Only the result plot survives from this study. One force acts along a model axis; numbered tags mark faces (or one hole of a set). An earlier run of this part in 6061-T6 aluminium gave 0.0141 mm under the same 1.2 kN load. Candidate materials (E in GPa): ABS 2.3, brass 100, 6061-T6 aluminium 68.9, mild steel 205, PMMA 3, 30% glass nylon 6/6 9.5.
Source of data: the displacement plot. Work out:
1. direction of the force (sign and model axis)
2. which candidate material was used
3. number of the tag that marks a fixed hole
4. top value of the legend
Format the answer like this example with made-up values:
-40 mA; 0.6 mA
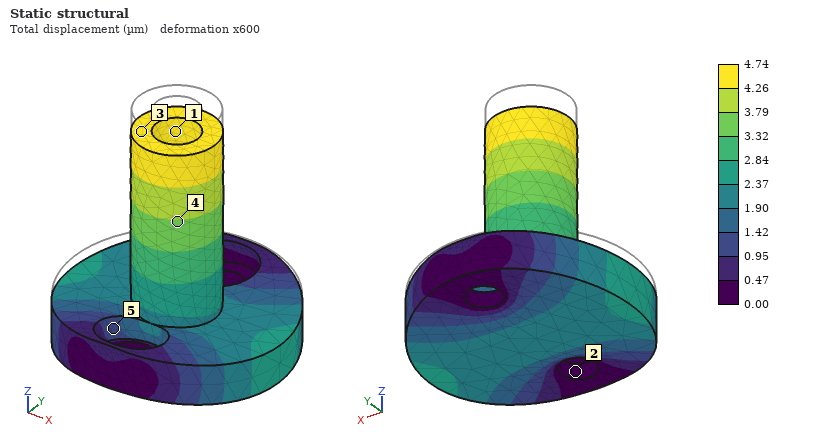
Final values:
-Z; mild steel; 2; 4.74 µm
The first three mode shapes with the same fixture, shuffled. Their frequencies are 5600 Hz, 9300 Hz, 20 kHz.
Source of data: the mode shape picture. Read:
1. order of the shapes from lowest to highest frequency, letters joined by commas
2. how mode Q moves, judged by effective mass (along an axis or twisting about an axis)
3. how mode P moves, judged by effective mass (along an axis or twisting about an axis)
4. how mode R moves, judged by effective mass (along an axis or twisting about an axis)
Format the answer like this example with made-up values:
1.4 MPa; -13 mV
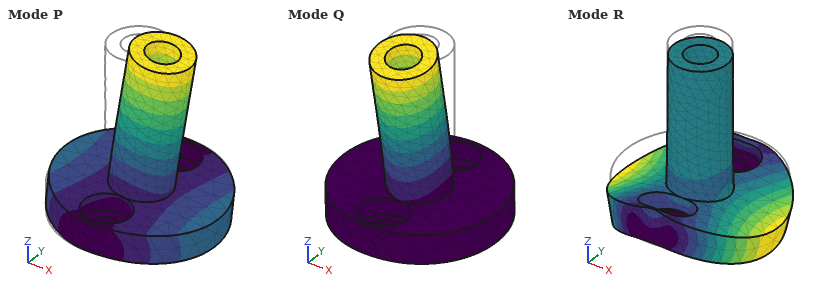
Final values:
P, Q, R; along Y; along X; along Z
